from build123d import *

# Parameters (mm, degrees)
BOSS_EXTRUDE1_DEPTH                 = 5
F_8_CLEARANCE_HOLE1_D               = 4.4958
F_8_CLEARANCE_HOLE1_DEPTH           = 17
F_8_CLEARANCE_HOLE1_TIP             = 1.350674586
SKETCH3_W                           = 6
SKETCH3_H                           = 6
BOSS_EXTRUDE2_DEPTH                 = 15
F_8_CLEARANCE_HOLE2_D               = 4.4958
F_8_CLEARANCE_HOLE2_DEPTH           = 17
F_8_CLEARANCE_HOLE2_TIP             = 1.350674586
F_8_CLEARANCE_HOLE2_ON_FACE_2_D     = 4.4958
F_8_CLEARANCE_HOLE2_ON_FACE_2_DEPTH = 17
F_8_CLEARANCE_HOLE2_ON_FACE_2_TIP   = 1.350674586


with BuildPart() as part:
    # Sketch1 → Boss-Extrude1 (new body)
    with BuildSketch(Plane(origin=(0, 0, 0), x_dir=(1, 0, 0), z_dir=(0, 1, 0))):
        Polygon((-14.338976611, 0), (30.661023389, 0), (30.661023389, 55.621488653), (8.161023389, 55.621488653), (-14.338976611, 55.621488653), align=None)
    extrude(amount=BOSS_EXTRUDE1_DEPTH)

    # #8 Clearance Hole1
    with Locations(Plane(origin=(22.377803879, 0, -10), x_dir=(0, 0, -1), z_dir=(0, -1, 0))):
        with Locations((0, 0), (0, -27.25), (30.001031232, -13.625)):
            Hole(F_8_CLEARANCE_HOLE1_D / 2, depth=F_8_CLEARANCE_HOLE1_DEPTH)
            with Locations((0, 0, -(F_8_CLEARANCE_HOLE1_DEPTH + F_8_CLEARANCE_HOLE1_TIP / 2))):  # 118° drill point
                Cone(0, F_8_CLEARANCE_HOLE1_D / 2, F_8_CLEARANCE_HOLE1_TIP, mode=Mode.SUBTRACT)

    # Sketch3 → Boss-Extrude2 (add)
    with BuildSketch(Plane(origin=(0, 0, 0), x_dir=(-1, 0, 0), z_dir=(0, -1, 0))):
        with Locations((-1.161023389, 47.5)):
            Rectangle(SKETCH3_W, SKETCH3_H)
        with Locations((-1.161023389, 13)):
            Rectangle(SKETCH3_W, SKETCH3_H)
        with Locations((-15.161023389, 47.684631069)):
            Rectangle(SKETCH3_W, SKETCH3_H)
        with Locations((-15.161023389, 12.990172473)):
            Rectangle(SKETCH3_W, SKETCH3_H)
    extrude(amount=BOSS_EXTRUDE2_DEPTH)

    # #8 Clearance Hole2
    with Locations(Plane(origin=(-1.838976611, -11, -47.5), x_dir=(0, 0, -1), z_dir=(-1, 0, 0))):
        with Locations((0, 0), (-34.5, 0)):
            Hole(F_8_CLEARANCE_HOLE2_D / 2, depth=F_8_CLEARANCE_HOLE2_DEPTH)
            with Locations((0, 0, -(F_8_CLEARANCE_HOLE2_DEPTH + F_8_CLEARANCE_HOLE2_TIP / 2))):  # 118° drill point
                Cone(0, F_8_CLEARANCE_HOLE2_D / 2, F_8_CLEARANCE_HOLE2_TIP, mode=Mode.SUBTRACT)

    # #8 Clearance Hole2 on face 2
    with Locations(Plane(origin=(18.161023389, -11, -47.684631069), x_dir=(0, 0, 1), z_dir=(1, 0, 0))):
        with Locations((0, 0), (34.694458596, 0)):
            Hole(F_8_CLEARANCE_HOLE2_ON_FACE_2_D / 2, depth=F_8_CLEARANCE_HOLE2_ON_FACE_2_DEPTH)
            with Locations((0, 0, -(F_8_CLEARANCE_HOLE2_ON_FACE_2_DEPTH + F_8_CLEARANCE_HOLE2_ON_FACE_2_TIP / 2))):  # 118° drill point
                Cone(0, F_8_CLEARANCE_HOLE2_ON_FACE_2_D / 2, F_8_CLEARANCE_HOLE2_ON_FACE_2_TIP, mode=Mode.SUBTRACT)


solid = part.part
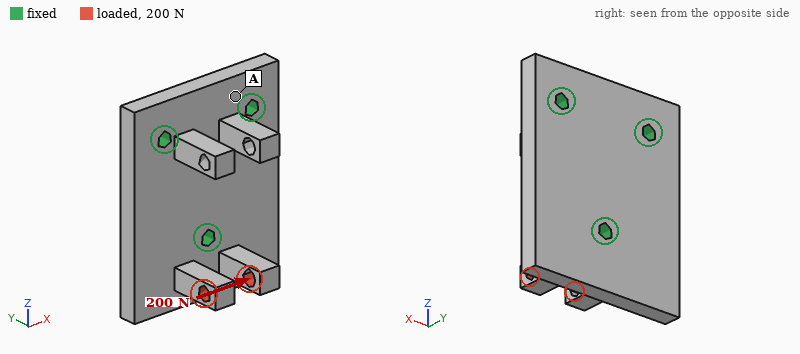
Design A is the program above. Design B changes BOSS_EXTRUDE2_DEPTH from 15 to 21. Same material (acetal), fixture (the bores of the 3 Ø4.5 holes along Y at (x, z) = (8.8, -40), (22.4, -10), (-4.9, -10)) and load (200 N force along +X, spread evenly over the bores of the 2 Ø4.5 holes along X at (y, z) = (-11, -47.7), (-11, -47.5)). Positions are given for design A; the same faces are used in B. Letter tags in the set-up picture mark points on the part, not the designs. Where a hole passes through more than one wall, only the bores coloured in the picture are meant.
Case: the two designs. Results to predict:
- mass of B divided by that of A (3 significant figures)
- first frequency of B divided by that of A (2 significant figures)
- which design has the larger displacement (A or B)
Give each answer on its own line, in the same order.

1.06
0.81
B
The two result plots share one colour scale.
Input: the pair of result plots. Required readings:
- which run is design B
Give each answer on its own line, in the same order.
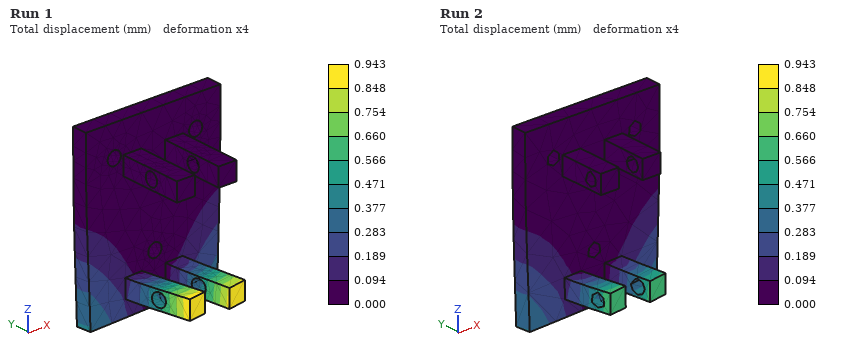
Run 1
